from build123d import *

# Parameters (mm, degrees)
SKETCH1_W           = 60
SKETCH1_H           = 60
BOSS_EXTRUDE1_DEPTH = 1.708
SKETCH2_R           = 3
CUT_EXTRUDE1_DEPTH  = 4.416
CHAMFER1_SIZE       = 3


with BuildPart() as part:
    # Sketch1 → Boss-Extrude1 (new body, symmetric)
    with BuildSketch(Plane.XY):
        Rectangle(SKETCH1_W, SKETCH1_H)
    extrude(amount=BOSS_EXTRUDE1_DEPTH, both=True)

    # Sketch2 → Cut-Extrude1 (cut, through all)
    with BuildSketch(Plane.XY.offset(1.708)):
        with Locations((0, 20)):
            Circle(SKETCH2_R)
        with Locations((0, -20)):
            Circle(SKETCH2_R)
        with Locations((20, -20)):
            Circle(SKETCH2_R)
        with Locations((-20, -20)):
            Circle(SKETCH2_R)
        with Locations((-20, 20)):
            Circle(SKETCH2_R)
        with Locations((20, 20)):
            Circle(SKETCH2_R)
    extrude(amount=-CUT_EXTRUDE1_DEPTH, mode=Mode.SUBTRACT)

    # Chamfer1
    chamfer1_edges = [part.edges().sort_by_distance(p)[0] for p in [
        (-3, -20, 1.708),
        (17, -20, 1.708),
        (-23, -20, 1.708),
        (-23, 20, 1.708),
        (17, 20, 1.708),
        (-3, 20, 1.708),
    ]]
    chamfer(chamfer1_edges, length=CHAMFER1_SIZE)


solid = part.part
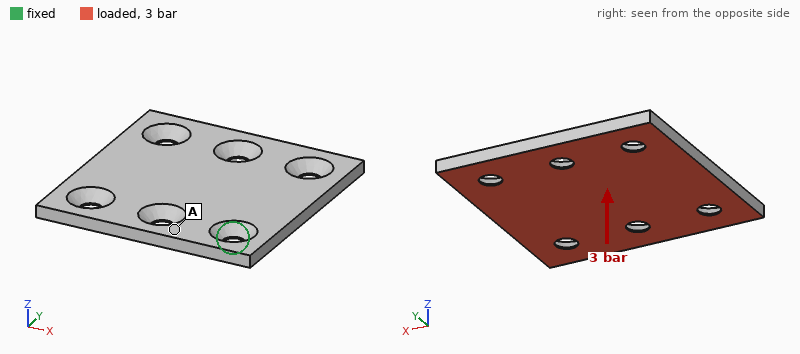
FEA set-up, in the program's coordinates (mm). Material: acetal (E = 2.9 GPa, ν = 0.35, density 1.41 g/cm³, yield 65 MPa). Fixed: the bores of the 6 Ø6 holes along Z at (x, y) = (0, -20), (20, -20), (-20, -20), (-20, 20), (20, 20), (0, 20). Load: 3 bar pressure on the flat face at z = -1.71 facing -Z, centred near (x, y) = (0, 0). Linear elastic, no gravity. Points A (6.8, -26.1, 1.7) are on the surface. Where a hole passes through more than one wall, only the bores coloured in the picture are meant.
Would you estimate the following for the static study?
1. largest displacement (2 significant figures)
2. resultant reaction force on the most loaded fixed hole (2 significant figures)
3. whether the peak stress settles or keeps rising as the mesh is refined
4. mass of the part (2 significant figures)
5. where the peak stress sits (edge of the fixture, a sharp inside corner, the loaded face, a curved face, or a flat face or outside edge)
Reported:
0.39 mm
230 N
keeps rising
16 g
edge of the fixture
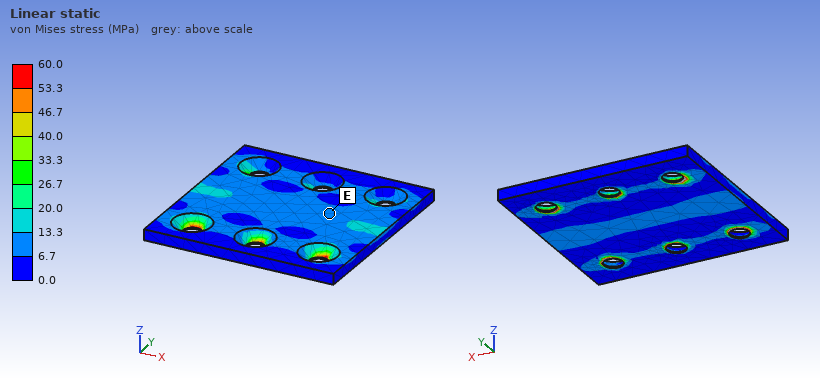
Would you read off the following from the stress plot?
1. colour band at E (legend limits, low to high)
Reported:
6.7 to 13.3 MPa
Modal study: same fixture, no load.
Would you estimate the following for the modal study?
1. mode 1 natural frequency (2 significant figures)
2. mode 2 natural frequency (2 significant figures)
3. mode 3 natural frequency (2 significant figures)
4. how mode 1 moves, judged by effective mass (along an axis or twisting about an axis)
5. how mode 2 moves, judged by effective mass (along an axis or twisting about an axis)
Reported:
2400 Hz
2600 Hz
3500 Hz
along Z
twisting about Y
